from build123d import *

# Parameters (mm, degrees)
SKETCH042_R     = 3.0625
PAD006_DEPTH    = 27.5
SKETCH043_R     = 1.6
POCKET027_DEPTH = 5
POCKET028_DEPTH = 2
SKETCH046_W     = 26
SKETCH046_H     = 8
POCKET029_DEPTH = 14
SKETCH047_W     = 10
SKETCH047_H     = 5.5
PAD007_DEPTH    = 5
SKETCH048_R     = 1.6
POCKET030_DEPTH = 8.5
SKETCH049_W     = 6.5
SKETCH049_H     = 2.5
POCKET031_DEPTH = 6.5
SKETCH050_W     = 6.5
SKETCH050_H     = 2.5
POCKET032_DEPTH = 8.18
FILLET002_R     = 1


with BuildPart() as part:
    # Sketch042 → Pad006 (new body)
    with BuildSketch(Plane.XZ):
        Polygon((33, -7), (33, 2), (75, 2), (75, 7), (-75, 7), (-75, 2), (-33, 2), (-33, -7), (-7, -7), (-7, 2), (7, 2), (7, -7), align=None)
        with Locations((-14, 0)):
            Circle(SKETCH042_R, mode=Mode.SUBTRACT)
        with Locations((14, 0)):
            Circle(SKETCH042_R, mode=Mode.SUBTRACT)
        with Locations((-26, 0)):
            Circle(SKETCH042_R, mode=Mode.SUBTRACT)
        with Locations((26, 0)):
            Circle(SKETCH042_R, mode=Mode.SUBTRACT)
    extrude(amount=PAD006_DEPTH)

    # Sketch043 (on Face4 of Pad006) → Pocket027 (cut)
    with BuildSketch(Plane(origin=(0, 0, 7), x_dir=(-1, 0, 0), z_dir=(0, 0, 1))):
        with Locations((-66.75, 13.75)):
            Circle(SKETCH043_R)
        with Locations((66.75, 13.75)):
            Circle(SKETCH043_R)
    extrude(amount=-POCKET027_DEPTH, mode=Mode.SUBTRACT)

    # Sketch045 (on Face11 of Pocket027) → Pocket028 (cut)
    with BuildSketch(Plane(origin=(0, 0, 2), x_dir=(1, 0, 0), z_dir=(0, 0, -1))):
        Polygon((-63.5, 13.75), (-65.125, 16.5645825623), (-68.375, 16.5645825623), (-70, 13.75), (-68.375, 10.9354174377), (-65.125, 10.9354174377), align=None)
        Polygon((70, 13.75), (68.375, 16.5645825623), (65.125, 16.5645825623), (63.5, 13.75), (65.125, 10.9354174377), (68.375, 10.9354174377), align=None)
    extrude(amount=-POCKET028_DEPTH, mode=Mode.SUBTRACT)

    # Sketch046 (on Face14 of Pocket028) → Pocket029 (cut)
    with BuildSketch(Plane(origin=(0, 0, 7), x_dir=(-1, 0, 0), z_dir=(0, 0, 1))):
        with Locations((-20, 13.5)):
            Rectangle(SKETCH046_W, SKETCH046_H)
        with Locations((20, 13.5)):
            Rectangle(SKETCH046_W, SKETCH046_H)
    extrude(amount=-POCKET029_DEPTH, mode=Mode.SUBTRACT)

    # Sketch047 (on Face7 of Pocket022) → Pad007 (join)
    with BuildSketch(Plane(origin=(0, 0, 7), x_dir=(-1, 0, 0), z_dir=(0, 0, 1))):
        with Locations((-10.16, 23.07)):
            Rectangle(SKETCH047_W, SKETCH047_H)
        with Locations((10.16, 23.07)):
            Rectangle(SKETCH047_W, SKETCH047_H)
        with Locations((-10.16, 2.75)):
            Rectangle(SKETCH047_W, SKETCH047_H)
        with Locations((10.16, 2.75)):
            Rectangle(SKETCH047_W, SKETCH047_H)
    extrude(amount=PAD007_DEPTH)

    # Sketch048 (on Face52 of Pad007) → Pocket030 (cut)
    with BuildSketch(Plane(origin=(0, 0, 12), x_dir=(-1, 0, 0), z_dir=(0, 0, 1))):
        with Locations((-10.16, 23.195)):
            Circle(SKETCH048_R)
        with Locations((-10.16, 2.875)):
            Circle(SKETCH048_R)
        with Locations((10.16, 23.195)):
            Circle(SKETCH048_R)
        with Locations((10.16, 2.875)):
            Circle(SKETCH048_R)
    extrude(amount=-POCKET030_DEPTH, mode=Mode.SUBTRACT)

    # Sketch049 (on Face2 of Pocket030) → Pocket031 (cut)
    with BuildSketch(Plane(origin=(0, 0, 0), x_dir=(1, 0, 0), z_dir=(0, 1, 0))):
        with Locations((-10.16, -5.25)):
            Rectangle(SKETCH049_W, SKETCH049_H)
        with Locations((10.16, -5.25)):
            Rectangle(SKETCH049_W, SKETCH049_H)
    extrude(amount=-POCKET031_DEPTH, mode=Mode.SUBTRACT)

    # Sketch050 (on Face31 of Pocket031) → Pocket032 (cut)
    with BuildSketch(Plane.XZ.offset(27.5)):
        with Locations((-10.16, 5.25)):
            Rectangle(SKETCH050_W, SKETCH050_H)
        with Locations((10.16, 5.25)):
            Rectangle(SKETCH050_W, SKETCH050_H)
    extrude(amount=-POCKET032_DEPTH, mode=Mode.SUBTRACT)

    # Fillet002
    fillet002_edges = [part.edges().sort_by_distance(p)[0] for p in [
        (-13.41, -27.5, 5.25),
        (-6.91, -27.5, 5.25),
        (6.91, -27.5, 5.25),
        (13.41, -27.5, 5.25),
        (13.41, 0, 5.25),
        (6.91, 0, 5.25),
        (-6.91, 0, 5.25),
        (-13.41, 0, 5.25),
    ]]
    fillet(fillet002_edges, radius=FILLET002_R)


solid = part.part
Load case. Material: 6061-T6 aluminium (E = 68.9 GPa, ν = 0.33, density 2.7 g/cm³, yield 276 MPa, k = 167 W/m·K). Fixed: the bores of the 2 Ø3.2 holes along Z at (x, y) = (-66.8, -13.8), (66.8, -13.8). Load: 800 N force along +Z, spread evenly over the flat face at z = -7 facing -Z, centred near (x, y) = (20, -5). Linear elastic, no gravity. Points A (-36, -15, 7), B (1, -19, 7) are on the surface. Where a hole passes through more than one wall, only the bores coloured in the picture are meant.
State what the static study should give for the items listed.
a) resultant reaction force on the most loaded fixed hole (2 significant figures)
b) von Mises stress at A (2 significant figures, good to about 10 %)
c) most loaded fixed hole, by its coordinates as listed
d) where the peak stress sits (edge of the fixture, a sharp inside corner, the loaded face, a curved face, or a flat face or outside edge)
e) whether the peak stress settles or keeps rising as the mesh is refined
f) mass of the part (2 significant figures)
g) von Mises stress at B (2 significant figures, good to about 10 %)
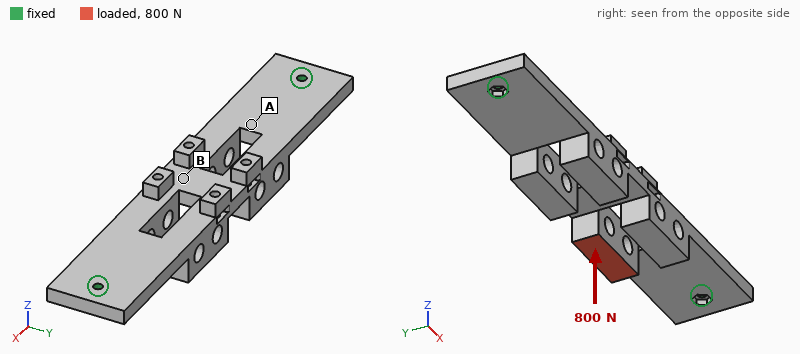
940 N
17 MPa
(66.8, -13.8)
edge of the fixture
keeps rising
69 g
81 MPa
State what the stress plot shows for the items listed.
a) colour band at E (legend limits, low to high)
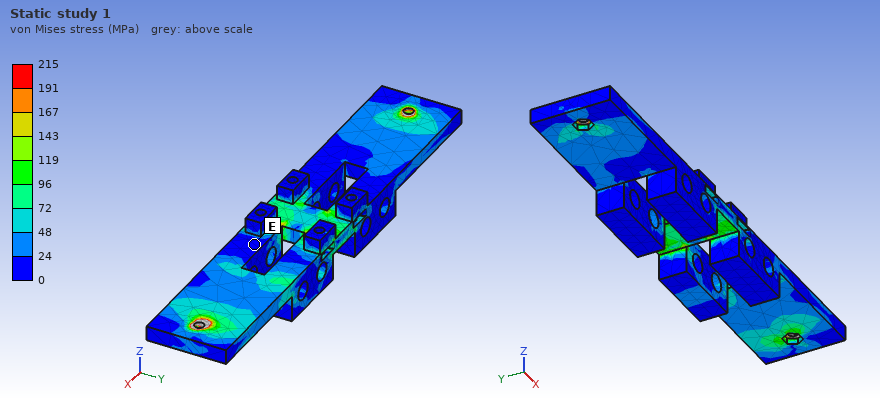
0 to 24 MPa
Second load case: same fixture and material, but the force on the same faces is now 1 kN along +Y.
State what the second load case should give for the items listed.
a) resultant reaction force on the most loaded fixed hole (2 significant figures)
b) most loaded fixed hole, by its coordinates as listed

660 N
(66.8, -13.8)
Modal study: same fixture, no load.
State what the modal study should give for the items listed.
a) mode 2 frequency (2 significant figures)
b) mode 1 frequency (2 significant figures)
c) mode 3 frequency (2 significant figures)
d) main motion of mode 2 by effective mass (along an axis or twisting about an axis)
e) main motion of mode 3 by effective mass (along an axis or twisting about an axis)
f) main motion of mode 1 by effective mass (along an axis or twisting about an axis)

2100 Hz
1100 Hz
2900 Hz
along Y
along Y
along Z
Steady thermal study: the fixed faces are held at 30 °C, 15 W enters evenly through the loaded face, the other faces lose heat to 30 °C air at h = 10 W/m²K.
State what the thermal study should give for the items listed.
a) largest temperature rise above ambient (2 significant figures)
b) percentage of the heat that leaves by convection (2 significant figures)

30 K
11 %
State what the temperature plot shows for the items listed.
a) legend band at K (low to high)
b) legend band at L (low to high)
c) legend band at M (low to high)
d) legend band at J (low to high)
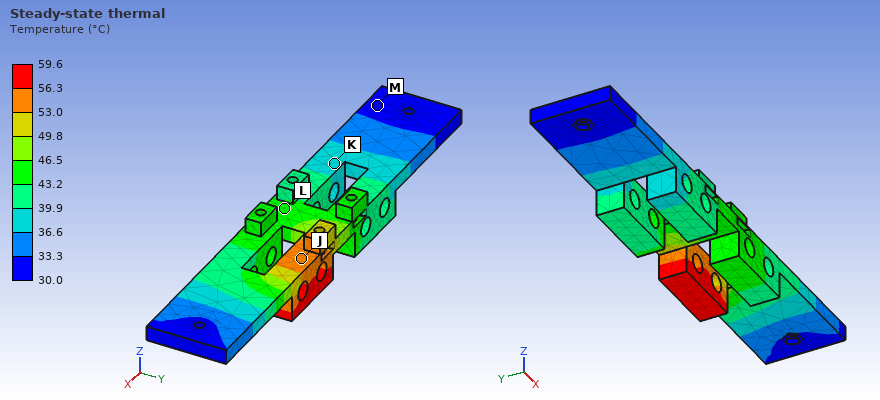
36.6 to 39.9 °C
43.2 to 46.5 °C
30.0 to 33.3 °C
53.0 to 56.3 °C
